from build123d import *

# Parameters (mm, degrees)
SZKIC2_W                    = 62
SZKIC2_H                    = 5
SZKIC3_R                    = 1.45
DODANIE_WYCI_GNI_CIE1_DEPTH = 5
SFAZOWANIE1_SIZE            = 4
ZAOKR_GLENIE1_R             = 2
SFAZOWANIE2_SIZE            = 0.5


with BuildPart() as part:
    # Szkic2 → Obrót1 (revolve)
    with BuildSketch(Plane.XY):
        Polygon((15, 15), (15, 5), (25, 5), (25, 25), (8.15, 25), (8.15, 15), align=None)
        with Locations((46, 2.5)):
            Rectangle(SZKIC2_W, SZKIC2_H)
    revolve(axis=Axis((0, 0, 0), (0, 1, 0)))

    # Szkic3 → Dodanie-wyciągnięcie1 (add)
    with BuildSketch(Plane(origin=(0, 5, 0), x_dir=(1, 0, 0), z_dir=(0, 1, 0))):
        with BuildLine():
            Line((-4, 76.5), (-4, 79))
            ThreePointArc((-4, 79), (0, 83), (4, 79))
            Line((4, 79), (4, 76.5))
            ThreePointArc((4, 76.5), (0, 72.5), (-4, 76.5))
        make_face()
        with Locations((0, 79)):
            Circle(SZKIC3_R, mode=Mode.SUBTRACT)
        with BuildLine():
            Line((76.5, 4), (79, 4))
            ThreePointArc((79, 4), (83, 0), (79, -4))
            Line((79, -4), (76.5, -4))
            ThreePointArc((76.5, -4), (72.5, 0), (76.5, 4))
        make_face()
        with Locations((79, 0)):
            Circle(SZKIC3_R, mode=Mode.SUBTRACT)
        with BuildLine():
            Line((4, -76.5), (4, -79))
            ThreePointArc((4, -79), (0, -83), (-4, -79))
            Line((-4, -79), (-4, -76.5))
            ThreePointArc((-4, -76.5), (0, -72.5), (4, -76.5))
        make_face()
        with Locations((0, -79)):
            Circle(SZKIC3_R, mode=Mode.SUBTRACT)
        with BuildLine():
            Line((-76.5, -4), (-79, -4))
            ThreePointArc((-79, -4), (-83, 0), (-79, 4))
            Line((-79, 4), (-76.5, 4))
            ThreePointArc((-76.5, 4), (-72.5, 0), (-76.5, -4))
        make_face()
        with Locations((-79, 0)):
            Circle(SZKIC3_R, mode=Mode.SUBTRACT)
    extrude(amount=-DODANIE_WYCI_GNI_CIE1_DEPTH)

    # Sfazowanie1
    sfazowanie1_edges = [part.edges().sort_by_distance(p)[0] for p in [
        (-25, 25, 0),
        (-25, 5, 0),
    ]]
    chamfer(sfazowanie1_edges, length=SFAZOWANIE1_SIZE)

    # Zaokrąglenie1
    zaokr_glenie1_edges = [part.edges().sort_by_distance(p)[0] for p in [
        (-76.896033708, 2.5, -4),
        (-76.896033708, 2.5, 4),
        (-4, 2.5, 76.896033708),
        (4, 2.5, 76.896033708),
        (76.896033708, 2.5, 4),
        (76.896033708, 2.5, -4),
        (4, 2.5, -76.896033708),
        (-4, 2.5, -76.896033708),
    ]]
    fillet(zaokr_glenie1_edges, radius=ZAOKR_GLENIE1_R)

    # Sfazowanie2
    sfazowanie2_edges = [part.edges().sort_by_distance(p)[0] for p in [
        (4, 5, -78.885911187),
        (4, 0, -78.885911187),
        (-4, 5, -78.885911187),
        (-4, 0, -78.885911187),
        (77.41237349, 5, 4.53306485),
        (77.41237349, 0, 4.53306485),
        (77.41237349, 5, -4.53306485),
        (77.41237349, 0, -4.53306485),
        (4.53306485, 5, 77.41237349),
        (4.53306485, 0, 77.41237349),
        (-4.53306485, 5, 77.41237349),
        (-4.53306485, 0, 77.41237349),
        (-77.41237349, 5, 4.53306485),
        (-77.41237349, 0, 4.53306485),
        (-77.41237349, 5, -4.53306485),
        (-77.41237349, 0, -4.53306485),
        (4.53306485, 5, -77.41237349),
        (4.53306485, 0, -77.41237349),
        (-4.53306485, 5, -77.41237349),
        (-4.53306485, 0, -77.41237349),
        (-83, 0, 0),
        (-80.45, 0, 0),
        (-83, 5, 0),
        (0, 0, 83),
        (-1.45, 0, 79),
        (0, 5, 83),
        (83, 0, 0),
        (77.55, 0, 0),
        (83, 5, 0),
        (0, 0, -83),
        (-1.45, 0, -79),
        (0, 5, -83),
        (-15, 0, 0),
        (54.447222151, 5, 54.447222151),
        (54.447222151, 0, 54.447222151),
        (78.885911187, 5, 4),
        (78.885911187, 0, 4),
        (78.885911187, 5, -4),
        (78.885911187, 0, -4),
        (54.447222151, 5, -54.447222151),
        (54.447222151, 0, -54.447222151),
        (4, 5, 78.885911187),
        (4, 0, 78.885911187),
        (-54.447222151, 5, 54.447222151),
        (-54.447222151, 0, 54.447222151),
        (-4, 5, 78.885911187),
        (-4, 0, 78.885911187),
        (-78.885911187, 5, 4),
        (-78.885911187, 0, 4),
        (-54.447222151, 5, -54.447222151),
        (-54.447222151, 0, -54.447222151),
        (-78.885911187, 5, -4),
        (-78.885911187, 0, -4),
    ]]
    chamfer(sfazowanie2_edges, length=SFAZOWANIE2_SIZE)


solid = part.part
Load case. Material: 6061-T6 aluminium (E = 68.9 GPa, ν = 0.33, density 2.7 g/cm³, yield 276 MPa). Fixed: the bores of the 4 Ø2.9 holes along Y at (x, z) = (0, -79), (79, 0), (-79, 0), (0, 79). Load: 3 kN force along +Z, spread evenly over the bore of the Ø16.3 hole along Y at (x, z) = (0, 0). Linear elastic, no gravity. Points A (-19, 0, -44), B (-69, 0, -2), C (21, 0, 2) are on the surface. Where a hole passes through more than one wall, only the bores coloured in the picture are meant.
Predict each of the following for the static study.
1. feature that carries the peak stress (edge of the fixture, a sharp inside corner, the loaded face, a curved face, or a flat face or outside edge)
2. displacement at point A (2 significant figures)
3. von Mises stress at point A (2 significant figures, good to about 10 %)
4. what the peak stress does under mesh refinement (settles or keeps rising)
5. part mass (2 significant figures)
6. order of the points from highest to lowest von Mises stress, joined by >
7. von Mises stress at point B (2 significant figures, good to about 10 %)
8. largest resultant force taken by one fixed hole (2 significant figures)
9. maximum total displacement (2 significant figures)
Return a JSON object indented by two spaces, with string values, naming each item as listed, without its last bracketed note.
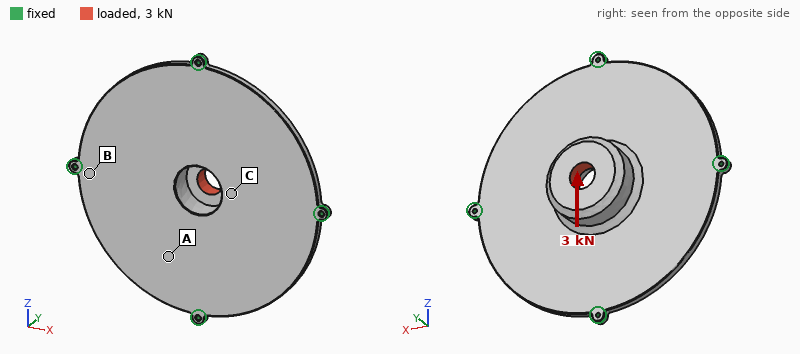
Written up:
{
  "feature that carries the peak stress": "edge of the fixture",
  "displacement at point A": "78 µm",
  "von Mises stress at point A": "18 MPa",
  "what the peak stress does under mesh refinement": "keeps rising",
  "part mass": "330 g",
  "order of the points from highest to lowest von Mises stress, joined by >": "A > B > C",
  "von Mises stress at point B": "12 MPa",
  "largest resultant force taken by one fixed hole": "1.1 kN",
  "maximum total displacement": "97 µm"
}
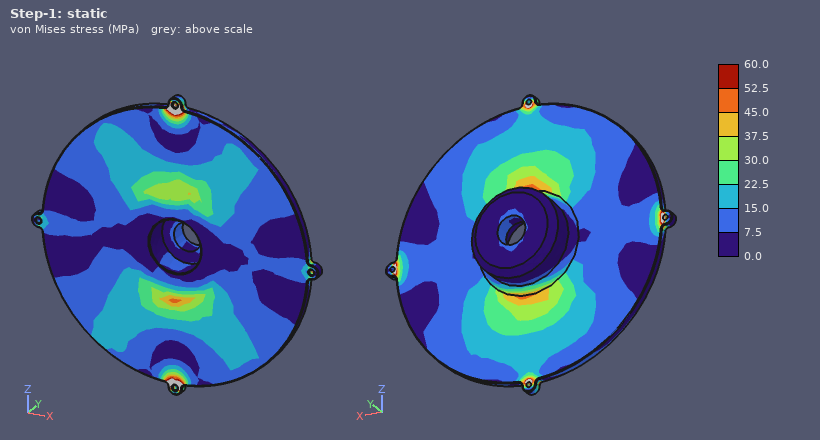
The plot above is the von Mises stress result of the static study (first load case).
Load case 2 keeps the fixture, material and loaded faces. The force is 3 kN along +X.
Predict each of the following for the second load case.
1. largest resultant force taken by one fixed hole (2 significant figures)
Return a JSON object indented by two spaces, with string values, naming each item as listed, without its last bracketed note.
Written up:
{
  "largest resultant force taken by one fixed hole": "1.1 kN"
}
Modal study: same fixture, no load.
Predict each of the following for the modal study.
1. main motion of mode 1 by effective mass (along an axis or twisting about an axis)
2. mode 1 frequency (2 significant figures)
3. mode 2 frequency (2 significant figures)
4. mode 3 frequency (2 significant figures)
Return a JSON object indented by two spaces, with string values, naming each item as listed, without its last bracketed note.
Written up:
{
  "main motion of mode 1 by effective mass": "along Y",
  "mode 1 frequency": "1000 Hz",
  "mode 2 frequency": "1700 Hz",
  "mode 3 frequency": "1700 Hz"
}
